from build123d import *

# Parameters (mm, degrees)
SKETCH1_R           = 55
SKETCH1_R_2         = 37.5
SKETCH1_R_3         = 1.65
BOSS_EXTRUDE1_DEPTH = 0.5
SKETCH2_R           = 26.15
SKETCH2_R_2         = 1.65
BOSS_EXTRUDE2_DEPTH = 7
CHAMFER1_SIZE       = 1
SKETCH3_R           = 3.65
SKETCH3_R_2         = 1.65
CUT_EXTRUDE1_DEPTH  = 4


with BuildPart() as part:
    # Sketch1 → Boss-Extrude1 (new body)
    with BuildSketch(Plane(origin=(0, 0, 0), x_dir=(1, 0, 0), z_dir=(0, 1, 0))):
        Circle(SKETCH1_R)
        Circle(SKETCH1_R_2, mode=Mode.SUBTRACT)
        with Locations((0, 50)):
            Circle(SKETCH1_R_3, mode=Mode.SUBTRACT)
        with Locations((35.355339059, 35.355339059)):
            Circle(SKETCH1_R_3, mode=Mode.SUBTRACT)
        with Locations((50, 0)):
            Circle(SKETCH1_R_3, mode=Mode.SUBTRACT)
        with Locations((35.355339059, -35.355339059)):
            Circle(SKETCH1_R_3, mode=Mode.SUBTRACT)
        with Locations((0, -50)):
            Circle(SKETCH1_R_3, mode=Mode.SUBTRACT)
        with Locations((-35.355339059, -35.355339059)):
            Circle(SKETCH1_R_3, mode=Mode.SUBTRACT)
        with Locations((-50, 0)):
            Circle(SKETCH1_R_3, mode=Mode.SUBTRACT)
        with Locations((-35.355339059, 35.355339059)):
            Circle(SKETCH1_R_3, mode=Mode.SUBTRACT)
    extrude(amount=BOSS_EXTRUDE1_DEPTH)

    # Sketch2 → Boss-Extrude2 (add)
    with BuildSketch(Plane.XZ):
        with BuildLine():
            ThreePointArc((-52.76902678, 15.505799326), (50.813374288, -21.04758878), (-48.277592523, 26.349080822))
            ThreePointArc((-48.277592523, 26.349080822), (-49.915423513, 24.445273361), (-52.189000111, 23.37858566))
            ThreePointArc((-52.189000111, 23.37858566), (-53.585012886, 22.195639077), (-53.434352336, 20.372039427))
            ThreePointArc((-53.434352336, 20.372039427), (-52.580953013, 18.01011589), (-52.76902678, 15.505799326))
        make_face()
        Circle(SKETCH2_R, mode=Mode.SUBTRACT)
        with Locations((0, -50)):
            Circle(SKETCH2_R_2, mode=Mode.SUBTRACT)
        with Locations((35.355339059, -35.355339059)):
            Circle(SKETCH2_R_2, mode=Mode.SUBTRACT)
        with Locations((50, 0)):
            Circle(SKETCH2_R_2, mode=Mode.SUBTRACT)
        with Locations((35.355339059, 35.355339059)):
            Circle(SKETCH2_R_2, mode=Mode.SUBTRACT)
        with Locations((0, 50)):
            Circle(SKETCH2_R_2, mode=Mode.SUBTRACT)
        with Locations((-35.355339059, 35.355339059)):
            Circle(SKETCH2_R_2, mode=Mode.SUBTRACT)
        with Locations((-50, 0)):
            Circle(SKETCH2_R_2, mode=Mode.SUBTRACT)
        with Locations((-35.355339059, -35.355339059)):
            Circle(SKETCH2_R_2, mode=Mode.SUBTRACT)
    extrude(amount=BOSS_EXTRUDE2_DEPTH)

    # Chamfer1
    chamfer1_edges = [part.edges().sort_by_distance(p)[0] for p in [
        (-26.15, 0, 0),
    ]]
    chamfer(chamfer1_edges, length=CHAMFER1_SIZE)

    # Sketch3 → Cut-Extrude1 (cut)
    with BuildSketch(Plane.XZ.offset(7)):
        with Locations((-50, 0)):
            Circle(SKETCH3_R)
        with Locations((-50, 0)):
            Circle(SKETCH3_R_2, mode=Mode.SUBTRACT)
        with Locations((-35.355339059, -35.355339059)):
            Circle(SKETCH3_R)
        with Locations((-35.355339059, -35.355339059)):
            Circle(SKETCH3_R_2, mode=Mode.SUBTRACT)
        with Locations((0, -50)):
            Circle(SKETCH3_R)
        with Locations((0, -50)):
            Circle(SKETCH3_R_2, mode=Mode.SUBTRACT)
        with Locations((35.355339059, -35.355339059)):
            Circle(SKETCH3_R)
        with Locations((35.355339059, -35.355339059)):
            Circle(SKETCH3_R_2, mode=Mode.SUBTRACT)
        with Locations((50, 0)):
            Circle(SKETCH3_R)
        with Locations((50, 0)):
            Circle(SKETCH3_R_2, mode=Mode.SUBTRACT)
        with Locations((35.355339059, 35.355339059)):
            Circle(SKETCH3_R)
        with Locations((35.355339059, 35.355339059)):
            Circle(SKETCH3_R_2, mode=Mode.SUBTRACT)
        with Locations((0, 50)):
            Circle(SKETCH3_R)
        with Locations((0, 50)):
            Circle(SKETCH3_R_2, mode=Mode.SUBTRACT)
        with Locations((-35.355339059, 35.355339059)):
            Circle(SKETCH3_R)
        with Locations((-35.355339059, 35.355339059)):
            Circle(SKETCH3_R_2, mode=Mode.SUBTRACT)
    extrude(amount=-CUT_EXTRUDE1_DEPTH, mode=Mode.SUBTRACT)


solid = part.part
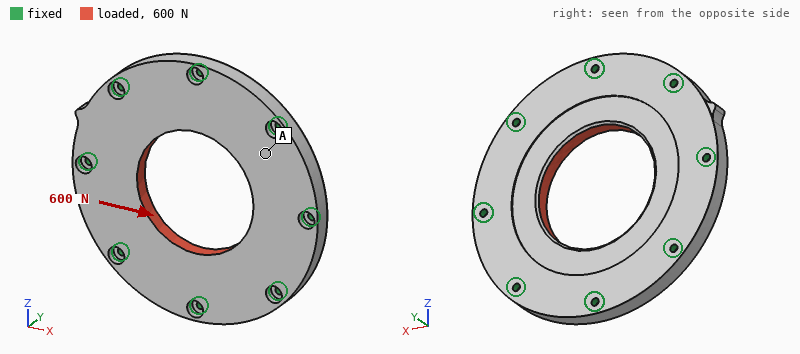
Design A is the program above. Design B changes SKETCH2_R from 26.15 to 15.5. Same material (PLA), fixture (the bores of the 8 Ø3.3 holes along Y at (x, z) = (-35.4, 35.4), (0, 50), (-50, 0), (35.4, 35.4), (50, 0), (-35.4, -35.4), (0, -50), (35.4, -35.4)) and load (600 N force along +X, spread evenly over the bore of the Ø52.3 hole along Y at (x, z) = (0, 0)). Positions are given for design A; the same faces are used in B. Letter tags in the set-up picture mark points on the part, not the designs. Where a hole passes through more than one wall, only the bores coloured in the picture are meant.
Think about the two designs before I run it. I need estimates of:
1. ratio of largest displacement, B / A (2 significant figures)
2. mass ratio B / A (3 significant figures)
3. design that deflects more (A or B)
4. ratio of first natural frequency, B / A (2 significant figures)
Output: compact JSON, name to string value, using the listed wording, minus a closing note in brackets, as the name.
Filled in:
{"ratio of largest displacement, B / A": "0.81", "mass ratio B / A": "1.19", "design that deflects more": "A", "ratio of first natural frequency, B / A": "0.77"}
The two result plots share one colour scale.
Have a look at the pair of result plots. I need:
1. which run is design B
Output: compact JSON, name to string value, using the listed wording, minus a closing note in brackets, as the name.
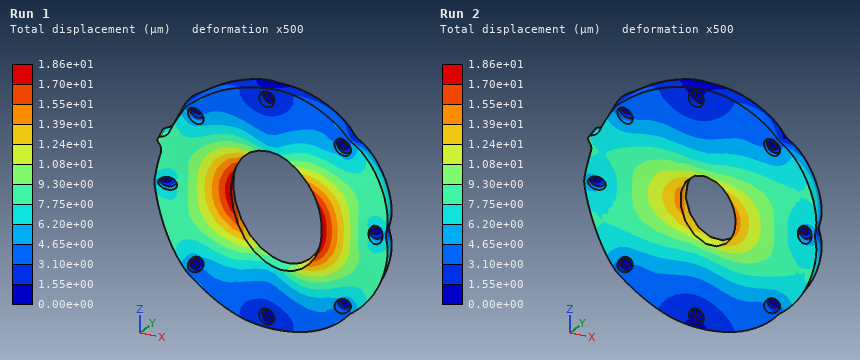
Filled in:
{"which run is design B": "Run 2"}
